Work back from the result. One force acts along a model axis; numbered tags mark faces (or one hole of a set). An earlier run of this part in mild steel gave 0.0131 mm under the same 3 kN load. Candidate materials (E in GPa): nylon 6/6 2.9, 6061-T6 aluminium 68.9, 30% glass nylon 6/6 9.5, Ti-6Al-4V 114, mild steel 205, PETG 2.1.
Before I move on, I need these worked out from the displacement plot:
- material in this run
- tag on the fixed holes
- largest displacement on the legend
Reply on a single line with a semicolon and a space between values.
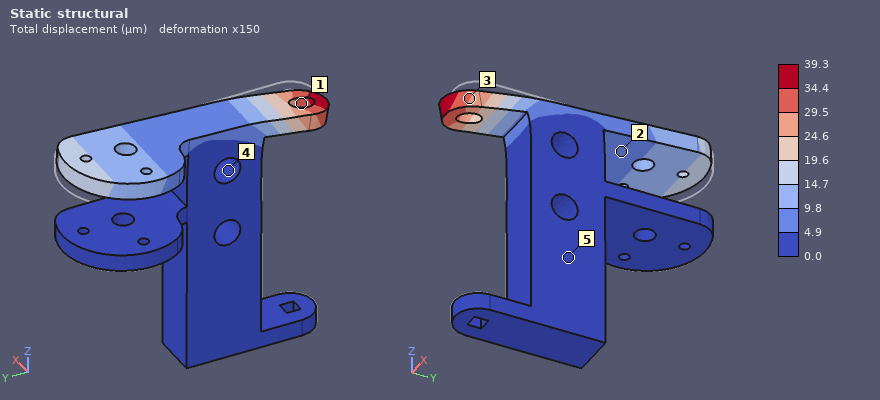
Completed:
6061-T6 aluminium; 4; 39.3 µm
